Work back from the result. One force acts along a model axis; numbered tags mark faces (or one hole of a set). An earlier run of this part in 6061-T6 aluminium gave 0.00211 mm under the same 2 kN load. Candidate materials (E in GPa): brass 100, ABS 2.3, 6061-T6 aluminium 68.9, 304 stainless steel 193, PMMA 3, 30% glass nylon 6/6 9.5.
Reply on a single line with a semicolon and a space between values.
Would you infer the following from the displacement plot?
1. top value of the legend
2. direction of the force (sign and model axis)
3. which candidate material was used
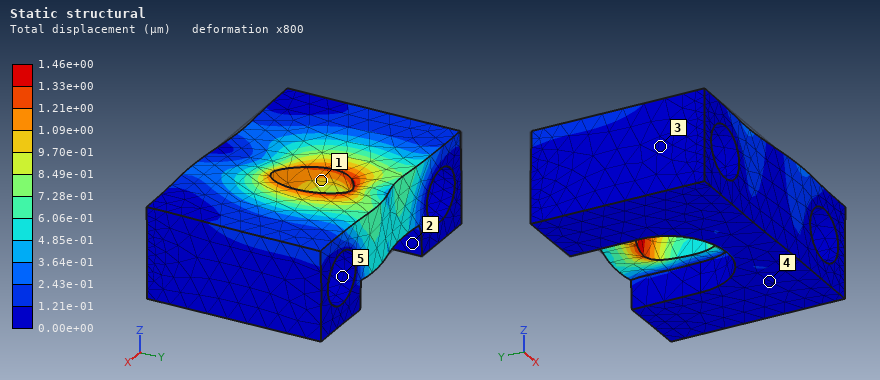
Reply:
1.46e+00 µm; +X; brass
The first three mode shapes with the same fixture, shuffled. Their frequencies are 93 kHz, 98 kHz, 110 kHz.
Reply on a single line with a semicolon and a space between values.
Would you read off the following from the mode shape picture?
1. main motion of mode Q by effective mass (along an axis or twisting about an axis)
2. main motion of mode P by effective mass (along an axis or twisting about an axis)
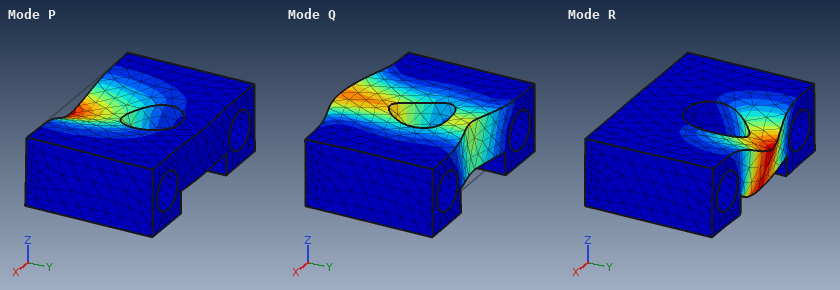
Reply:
along Y; along Z
